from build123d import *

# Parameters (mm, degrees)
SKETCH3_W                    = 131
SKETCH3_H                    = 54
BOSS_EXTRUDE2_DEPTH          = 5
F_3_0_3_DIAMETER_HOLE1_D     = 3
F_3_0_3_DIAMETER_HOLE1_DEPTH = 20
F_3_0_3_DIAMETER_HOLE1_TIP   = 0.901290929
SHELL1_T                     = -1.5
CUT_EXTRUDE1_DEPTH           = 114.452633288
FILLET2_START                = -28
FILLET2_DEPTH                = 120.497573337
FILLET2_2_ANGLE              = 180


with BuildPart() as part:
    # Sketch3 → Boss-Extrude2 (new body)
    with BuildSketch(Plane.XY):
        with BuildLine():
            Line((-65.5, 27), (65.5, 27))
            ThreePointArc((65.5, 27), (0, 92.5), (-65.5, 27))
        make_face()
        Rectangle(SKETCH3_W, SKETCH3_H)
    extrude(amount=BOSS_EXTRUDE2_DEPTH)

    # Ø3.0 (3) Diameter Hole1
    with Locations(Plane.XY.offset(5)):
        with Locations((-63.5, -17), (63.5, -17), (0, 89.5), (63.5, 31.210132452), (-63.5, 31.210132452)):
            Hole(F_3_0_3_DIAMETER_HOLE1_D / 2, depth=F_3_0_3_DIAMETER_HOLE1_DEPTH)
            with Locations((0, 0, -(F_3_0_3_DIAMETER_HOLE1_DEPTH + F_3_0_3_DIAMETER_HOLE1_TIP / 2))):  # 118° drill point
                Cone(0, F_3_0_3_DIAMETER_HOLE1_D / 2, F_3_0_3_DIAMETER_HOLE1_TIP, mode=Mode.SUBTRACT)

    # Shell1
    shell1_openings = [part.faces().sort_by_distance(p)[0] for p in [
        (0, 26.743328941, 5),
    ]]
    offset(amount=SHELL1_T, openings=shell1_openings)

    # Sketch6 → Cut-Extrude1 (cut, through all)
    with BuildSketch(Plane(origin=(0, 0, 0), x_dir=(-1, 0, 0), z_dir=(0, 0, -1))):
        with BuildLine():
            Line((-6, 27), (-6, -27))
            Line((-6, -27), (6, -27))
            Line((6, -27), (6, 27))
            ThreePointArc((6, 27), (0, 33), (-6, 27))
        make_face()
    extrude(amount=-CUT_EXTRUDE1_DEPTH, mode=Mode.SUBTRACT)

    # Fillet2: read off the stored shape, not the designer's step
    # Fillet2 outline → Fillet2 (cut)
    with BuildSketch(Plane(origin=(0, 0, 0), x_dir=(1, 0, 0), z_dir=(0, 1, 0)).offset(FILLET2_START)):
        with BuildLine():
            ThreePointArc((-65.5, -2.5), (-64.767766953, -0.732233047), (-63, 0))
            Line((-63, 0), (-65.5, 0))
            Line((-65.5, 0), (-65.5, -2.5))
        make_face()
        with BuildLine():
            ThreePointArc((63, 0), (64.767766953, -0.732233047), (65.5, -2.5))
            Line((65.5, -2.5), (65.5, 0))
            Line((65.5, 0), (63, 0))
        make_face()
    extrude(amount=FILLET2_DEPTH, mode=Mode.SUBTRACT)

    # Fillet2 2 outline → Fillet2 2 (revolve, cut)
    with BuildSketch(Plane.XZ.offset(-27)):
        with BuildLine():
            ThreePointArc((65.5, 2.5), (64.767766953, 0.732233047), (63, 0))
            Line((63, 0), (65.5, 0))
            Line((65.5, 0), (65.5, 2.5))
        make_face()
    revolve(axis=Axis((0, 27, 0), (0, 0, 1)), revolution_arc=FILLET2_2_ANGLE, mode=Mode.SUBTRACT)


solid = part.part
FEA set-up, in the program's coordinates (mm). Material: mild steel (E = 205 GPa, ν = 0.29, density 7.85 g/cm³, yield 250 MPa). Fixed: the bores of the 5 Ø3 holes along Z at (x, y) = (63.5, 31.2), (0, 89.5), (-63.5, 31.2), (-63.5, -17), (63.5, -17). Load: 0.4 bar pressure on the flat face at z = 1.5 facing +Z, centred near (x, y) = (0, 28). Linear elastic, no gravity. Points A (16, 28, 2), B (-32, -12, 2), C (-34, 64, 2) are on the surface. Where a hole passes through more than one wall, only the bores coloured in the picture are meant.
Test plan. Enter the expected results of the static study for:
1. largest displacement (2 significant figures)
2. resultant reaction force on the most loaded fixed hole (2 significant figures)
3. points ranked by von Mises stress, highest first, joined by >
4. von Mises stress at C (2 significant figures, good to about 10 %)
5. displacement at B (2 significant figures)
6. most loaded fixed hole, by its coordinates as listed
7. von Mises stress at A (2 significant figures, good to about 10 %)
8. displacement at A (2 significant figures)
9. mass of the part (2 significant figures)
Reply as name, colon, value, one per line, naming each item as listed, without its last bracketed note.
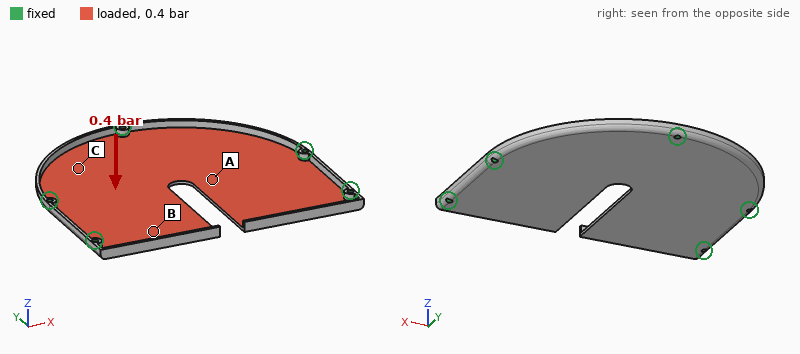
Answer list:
largest displacement: 0.49 mm
resultant reaction force on the most loaded fixed hole: 130 N
points ranked by von Mises stress, highest first, joined by >: A > C > B
von Mises stress at C: 28 MPa
displacement at B: 0.23 mm
most loaded fixed hole, by its coordinates as listed: (0, 89.5)
von Mises stress at A: 44 MPa
displacement at A: 0.35 mm
mass of the part: 170 g
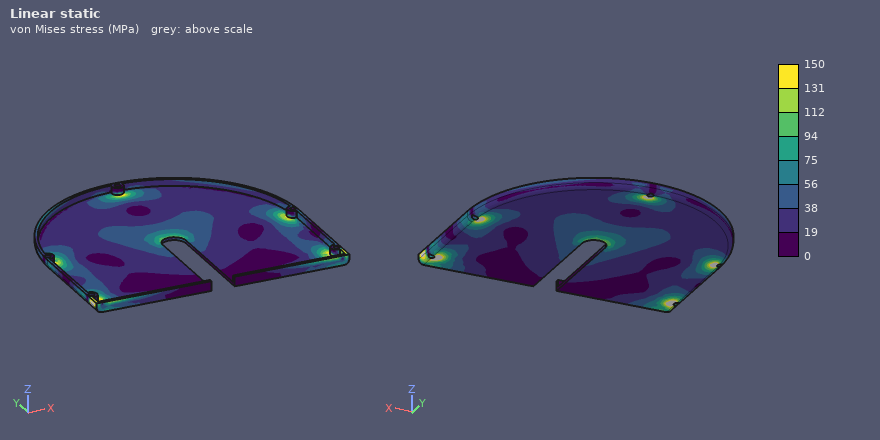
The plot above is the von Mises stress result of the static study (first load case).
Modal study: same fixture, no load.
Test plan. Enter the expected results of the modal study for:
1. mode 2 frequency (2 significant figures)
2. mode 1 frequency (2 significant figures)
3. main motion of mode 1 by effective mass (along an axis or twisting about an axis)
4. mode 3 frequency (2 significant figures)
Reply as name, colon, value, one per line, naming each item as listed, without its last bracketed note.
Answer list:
mode 2 frequency: 710 Hz
mode 1 frequency: 530 Hz
main motion of mode 1 by effective mass: along Z
mode 3 frequency: 980 Hz
